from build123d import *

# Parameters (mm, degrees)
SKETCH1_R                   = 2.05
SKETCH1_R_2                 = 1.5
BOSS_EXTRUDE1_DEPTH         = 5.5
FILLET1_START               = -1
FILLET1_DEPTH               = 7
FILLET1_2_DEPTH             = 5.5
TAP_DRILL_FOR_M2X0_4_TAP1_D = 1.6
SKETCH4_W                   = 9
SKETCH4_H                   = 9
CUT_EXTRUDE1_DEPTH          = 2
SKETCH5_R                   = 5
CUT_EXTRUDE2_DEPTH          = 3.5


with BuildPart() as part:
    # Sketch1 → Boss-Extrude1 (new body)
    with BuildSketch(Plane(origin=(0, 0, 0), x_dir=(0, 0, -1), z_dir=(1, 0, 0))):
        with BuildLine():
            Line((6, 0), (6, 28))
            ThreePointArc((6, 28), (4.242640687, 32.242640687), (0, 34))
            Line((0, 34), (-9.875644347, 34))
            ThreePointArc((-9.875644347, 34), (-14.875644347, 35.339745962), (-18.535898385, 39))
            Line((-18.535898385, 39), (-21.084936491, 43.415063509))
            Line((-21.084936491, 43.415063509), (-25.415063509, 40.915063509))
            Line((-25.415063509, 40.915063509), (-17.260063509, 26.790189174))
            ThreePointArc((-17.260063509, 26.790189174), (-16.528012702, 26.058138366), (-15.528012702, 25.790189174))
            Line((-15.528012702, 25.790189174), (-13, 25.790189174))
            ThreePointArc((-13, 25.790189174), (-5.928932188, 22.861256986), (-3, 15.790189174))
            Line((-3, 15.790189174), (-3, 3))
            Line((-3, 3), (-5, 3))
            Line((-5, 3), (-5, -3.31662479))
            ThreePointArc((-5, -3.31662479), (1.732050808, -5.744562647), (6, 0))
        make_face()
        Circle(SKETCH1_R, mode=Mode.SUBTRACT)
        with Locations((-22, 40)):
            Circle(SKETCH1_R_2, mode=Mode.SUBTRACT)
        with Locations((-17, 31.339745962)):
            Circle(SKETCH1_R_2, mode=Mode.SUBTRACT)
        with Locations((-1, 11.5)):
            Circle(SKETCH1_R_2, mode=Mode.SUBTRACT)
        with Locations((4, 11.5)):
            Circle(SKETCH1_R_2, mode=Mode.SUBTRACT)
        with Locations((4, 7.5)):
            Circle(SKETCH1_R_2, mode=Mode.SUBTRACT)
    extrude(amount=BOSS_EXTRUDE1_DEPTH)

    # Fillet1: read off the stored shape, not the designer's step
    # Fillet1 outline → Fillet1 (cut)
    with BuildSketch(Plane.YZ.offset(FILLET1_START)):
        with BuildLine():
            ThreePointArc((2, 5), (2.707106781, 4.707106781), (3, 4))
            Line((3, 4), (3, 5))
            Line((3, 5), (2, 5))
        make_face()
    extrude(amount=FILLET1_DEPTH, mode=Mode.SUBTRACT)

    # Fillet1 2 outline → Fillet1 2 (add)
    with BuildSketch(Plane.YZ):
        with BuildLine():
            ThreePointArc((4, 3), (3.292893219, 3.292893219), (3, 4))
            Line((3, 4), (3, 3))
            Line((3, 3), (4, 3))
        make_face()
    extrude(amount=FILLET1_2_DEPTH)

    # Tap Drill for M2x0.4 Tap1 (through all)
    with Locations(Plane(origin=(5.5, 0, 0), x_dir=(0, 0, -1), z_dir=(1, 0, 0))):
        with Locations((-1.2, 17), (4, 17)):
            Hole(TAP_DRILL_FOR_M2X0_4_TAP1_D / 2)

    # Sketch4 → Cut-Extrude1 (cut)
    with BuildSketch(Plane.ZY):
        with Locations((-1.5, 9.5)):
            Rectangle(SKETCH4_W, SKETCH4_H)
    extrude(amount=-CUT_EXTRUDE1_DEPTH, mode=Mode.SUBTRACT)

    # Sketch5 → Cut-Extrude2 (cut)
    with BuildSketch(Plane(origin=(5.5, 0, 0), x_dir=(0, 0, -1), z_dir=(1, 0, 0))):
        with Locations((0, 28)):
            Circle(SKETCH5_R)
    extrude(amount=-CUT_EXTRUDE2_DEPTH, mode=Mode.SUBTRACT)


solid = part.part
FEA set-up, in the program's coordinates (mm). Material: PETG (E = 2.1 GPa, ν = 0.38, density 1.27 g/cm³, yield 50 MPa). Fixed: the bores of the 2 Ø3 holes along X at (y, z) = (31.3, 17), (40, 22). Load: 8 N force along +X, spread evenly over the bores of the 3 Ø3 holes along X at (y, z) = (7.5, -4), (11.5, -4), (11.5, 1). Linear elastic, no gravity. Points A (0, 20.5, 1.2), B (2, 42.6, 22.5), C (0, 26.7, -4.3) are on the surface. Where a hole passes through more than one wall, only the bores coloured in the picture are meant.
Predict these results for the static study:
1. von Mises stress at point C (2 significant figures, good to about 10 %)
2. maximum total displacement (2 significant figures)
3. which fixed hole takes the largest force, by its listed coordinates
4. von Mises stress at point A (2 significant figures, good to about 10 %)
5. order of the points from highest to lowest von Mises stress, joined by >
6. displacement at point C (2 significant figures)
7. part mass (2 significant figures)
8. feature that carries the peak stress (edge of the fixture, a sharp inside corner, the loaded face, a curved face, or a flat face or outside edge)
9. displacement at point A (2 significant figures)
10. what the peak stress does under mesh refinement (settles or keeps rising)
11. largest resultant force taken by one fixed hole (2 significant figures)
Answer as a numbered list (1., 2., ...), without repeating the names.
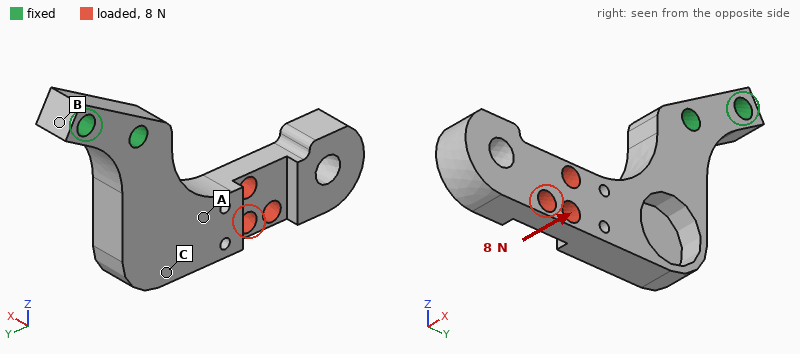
1. 1.6 MPa
2. 0.68 mm
3. (31.3, 17)
4. 2.3 MPa
5. A > C > B
6. 0.12 mm
7. 3.1 g
8. edge of the fixture
9. 0.17 mm
10. keeps rising
11. 11 N
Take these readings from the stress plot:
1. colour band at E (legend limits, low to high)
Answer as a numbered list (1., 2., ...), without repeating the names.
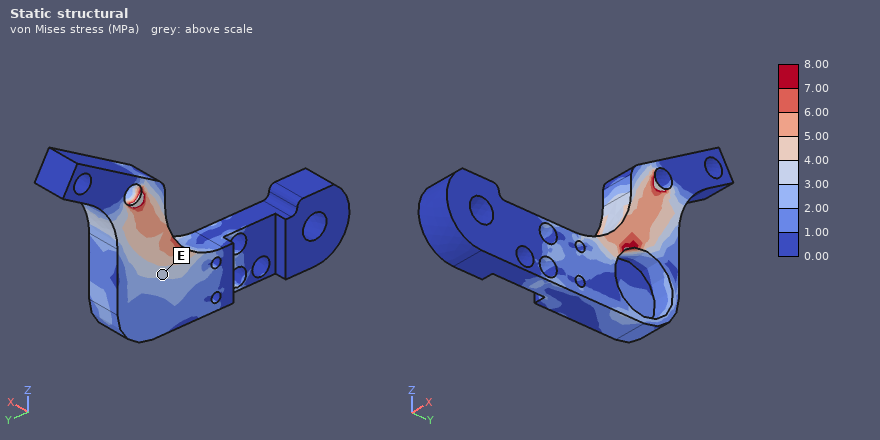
1. 3.00 to 4.00 MPa
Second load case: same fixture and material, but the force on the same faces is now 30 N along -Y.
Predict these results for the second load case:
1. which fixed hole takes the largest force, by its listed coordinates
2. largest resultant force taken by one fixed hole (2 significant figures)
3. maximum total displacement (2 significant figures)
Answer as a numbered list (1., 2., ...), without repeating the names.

1. (31.3, 17)
2. 37 N
3. 0.62 mm
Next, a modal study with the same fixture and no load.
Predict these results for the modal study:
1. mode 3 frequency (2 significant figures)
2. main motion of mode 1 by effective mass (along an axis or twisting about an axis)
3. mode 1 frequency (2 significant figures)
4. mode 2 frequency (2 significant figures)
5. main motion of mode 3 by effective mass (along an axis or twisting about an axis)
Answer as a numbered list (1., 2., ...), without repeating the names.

1. 1500 Hz
2. along X
3. 480 Hz
4. 770 Hz
5. along X
